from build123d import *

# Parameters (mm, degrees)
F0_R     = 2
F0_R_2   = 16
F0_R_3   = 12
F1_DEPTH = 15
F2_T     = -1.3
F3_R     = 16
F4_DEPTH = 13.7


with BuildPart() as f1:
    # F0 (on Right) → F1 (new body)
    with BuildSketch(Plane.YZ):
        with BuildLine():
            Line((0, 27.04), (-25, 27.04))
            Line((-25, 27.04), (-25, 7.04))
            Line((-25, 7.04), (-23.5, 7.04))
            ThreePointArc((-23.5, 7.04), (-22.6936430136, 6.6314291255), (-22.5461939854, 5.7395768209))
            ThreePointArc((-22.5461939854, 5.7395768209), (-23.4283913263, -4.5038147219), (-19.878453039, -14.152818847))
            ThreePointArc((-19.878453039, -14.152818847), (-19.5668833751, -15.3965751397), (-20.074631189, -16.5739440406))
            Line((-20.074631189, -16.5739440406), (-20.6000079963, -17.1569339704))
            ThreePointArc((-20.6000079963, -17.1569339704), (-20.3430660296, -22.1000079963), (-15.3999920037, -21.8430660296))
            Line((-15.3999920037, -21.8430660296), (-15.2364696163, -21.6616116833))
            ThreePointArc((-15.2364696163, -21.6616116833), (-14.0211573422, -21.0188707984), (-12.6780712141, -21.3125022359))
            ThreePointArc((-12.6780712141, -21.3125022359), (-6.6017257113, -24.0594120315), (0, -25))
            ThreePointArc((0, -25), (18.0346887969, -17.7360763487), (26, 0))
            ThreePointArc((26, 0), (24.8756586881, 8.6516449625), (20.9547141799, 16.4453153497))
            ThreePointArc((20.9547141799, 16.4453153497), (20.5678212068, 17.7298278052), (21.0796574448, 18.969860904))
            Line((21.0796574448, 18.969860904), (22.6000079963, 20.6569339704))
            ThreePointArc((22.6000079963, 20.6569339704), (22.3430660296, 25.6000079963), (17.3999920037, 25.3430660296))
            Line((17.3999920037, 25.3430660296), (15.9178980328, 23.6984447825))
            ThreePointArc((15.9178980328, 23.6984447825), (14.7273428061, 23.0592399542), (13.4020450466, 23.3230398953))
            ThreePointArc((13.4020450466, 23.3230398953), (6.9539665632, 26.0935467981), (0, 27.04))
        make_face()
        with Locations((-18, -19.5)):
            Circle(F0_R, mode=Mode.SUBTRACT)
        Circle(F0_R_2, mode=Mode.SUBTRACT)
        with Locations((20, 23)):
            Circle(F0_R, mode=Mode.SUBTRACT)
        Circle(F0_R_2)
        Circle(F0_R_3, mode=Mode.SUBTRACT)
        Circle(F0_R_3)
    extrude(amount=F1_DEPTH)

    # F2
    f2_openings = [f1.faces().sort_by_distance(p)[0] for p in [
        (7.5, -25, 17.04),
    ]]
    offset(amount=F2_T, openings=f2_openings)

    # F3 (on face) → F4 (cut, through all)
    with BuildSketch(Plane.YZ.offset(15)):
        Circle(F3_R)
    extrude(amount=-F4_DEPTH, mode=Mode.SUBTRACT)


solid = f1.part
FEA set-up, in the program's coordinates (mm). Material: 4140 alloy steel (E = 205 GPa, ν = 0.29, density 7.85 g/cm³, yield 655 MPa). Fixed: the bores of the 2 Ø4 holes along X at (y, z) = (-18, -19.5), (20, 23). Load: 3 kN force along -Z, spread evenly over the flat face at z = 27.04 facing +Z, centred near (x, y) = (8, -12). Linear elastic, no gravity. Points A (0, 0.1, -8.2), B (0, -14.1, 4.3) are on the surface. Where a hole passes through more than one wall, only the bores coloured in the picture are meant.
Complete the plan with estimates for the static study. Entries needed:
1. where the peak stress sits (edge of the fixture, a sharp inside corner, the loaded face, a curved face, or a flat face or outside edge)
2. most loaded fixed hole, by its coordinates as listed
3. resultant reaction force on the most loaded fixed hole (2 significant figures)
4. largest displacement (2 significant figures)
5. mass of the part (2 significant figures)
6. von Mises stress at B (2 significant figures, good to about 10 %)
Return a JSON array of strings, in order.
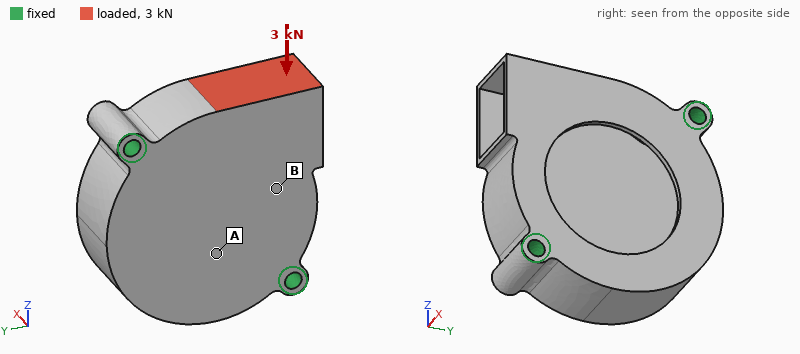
["the loaded face", "(-18, -19.5)", "2.2 kN", "71 µm", "61 g", "71 MPa"]
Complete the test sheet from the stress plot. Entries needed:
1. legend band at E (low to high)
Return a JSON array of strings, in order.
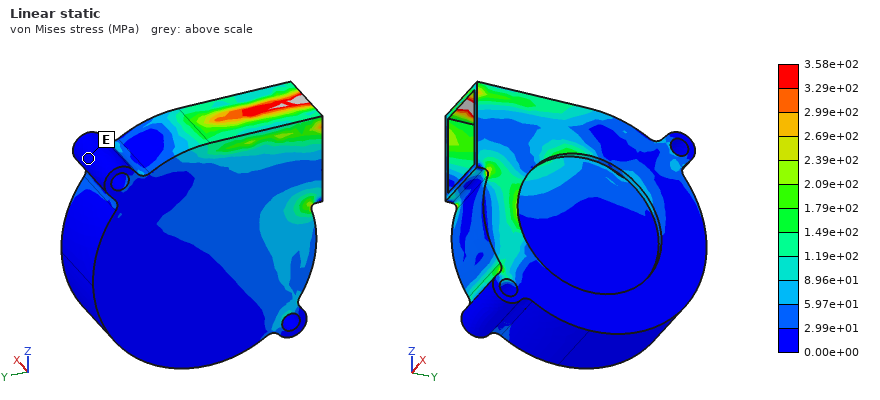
["0.00e+00 to 2.99e+01 MPa"]
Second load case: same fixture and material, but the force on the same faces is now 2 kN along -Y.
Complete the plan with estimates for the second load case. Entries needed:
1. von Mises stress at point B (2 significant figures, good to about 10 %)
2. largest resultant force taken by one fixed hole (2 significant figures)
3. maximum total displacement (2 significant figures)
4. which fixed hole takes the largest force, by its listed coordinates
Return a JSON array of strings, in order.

["9.9 MPa", "1.9 kN", "16 µm", "(20, 23)"]
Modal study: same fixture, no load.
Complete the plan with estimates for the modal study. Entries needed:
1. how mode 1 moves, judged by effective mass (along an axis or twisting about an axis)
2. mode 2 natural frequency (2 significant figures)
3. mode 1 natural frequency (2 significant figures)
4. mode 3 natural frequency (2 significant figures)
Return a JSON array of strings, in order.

["along X", "6200 Hz", "4500 Hz", "8100 Hz"]
